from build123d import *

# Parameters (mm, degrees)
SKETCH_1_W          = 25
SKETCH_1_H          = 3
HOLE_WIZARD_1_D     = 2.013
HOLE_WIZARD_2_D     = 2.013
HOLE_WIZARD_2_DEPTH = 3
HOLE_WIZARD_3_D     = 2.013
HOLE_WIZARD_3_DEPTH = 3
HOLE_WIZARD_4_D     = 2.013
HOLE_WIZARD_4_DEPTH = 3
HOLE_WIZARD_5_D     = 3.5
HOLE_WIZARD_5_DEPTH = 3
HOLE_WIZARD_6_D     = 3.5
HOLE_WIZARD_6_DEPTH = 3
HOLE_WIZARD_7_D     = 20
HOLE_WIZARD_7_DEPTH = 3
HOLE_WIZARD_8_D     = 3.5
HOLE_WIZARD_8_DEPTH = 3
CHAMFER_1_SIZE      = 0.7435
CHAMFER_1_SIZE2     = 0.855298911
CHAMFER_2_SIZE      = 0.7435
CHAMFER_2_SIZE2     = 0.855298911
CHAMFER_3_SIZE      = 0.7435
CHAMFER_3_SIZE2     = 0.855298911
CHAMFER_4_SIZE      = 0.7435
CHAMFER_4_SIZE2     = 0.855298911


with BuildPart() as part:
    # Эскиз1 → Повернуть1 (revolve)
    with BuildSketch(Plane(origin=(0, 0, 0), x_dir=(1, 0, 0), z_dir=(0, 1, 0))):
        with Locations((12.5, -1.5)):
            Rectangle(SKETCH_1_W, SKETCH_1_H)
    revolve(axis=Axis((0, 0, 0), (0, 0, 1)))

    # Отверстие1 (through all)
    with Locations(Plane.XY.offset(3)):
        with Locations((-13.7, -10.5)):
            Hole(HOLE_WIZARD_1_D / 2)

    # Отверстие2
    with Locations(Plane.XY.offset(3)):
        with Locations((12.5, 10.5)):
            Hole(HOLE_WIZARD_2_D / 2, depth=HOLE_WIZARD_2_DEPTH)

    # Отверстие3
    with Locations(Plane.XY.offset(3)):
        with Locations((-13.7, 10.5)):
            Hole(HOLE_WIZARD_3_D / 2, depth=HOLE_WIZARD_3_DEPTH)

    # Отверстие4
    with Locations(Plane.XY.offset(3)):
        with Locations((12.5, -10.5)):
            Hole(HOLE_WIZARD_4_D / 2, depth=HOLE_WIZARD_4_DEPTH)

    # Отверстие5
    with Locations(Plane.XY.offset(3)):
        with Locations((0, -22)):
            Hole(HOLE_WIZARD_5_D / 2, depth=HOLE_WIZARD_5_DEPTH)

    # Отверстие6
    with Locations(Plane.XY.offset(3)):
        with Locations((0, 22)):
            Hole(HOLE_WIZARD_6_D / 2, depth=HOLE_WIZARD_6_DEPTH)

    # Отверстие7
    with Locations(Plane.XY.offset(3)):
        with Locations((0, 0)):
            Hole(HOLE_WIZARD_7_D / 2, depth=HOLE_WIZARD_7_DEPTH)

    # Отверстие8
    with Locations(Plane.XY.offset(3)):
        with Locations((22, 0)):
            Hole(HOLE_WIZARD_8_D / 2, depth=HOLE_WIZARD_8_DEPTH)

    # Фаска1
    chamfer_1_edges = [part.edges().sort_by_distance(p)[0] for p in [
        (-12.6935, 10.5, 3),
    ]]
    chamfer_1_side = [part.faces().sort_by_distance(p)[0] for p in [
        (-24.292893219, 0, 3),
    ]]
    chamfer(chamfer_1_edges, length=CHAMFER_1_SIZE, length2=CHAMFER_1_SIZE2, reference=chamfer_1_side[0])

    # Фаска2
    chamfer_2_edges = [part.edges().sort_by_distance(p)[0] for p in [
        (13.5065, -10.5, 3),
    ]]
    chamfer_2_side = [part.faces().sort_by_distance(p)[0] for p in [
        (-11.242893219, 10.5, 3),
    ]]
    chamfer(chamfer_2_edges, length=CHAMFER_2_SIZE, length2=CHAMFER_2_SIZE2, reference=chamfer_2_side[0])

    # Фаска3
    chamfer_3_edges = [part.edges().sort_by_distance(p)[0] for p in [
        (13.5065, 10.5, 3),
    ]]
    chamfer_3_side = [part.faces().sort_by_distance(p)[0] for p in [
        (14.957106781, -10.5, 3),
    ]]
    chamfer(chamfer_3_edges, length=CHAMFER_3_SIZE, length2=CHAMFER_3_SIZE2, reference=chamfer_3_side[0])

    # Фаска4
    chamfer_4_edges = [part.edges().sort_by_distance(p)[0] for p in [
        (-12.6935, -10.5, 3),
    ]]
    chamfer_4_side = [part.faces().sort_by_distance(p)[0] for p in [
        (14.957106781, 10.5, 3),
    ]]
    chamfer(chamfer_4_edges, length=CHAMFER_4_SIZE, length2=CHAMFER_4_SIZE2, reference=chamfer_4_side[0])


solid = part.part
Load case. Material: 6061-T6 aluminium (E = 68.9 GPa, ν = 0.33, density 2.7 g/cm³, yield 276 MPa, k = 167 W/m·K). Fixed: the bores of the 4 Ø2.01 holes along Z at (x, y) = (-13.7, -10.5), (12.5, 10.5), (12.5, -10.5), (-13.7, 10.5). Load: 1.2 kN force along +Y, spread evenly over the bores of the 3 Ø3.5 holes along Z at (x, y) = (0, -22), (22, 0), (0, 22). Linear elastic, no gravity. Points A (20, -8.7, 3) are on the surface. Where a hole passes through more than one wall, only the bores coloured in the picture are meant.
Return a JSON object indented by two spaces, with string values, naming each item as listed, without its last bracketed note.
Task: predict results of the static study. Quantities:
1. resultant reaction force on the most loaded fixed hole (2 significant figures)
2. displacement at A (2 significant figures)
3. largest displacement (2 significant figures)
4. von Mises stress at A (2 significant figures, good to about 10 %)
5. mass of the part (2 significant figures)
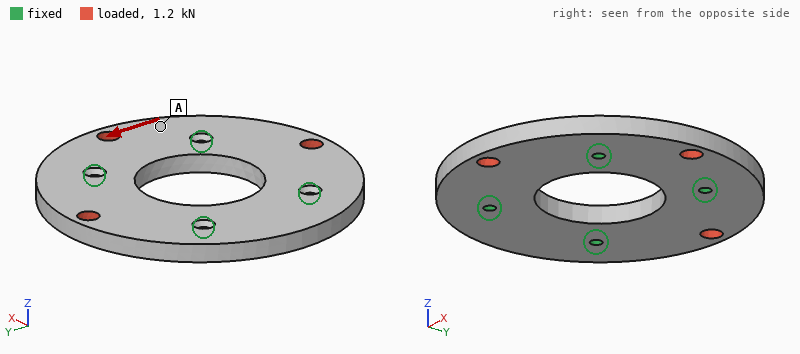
{
  "resultant reaction force on the most loaded fixed hole": "460 N",
  "displacement at A": "2.0 µm",
  "largest displacement": "5.4 µm",
  "von Mises stress at A": "6.0 MPa",
  "mass of the part": "13 g"
}
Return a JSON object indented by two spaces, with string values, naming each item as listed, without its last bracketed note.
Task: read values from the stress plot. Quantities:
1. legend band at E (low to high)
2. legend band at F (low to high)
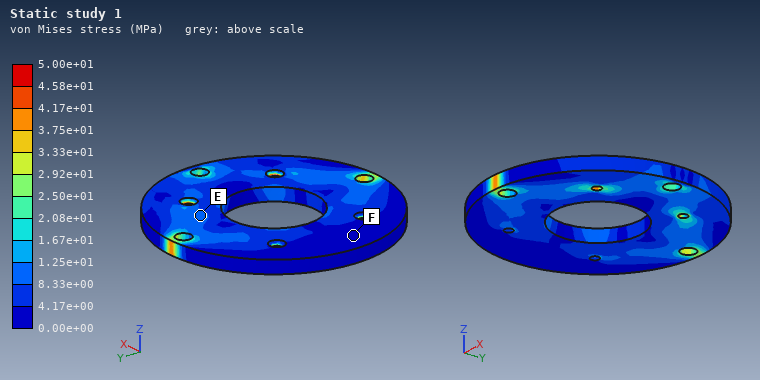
{
  "legend band at E": "8.33e+00 to 1.25e+01 MPa",
  "legend band at F": "0.00e+00 to 4.17e+00 MPa"
}
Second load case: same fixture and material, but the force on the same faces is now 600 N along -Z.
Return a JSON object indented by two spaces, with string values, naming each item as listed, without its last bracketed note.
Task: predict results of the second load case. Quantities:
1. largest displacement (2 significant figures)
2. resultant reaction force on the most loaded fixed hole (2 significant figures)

{
  "largest displacement": "72 µm",
  "resultant reaction force on the most loaded fixed hole": "220 N"
}
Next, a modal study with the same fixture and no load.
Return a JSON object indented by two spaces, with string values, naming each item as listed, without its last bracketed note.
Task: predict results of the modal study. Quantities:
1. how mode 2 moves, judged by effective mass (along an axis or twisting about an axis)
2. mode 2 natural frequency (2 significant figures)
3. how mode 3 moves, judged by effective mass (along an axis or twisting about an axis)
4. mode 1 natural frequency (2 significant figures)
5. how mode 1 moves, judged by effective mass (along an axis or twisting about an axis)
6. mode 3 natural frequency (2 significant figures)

{
  "how mode 2 moves, judged by effective mass": "twisting about X",
  "mode 2 natural frequency": "9700 Hz",
  "how mode 3 moves, judged by effective mass": "along Z",
  "mode 1 natural frequency": "9000 Hz",
  "how mode 1 moves, judged by effective mass": "along Z",
  "mode 3 natural frequency": "14 kHz"
}
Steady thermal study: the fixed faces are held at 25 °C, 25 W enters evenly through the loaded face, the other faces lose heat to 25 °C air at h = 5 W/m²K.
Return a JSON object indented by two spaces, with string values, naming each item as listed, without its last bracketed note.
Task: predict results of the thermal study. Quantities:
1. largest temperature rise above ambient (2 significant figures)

{
  "largest temperature rise above ambient": "17 K"
}
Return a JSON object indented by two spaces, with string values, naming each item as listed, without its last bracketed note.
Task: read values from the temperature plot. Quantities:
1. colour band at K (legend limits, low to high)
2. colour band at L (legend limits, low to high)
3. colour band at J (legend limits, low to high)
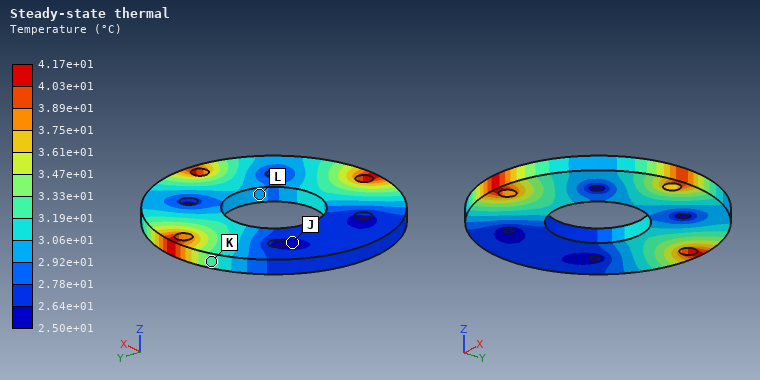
{
  "colour band at K": "3.19e+01 to 3.33e+01 °C",
  "colour band at L": "2.92e+01 to 3.06e+01 °C",
  "colour band at J": "2.50e+01 to 2.64e+01 °C"
}
